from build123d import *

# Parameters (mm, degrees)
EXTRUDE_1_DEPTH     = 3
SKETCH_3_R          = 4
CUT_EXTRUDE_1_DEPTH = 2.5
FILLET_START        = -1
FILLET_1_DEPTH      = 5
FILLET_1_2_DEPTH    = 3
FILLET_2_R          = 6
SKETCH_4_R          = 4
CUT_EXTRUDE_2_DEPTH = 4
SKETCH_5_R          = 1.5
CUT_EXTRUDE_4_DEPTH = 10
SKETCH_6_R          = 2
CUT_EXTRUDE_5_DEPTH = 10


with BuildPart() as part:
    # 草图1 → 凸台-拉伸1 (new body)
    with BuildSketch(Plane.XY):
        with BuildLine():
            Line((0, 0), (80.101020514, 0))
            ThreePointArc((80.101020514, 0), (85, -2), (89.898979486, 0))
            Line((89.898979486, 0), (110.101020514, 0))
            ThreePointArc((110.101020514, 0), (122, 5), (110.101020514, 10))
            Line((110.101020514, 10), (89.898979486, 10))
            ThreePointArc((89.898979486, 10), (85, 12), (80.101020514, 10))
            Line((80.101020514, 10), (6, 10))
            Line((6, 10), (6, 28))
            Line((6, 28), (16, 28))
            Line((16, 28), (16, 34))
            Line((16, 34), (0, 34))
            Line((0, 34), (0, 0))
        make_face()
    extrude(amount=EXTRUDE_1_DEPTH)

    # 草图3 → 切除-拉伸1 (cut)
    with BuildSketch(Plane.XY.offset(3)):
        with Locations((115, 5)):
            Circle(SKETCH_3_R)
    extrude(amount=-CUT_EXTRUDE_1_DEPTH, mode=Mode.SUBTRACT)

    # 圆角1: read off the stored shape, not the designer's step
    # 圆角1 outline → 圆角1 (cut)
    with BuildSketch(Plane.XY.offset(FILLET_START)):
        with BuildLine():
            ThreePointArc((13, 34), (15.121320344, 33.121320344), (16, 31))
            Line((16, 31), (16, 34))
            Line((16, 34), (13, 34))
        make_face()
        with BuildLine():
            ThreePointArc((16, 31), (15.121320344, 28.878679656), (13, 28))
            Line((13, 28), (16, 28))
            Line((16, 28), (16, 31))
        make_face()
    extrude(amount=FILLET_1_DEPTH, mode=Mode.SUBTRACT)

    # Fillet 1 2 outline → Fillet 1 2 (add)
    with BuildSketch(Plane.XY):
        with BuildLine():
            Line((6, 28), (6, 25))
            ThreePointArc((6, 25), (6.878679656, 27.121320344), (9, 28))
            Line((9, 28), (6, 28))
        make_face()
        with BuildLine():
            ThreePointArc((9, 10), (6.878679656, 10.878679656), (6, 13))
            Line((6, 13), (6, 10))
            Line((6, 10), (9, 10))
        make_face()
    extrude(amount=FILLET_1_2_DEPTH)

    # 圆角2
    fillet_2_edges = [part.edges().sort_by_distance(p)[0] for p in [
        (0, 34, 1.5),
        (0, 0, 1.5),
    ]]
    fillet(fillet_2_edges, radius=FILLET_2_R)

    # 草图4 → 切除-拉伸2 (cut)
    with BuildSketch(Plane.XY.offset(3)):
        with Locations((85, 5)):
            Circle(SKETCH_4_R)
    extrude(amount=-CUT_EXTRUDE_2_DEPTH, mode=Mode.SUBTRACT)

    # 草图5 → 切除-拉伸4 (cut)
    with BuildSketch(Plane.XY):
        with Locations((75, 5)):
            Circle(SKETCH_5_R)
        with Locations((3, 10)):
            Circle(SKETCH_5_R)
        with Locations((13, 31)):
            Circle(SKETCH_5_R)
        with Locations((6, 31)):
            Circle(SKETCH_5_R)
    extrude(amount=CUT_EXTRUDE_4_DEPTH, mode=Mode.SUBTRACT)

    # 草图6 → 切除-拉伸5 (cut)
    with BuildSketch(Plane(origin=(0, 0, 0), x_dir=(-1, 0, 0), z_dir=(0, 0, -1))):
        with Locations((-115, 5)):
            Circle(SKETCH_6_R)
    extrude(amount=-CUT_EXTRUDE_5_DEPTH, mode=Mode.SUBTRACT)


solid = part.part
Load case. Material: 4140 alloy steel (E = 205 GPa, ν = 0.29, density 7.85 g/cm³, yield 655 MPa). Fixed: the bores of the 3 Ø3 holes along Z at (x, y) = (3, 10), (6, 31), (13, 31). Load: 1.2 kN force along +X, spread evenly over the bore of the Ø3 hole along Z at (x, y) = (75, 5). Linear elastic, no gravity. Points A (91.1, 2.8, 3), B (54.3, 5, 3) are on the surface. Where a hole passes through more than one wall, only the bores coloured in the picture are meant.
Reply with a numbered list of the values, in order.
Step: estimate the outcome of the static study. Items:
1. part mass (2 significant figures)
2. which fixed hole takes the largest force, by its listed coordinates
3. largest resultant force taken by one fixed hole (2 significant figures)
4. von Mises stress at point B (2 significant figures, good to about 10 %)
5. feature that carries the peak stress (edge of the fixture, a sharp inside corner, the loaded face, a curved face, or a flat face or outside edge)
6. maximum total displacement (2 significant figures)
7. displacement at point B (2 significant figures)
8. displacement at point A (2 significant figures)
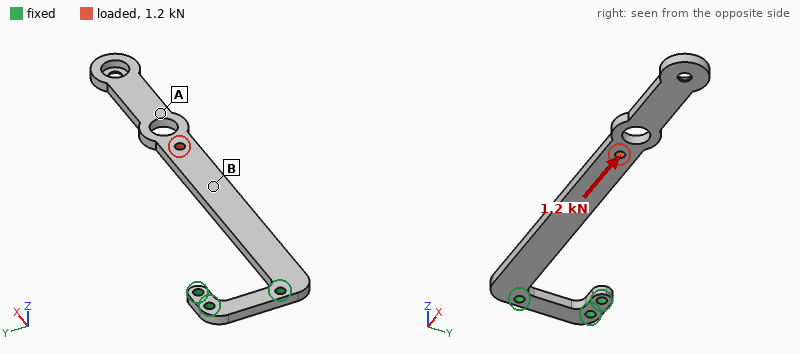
1. 31 g
2. (3, 10)
3. 1.3 kN
4. 40 MPa
5. edge of the fixture
6. 0.17 mm
7. 0.072 mm
8. 0.12 mm
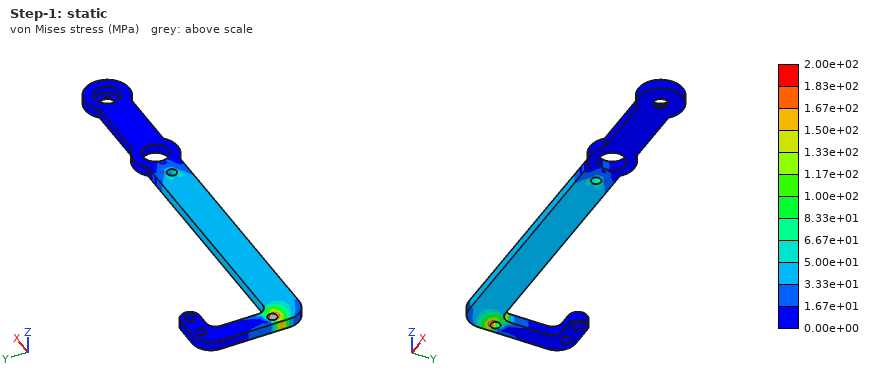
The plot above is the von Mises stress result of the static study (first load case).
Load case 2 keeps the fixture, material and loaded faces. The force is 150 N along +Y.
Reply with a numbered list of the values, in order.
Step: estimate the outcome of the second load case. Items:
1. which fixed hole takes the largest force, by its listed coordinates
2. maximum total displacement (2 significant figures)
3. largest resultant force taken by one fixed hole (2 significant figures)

1. (3, 10)
2. 0.98 mm
3. 180 N
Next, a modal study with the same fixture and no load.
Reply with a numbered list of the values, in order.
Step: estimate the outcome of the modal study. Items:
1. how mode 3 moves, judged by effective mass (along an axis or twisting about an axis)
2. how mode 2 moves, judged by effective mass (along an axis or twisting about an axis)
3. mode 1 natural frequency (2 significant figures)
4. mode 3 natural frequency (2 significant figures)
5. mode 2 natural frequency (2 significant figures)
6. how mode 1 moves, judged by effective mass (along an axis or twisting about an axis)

1. along Z
2. along Y
3. 180 Hz
4. 1100 Hz
5. 530 Hz
6. along Z
